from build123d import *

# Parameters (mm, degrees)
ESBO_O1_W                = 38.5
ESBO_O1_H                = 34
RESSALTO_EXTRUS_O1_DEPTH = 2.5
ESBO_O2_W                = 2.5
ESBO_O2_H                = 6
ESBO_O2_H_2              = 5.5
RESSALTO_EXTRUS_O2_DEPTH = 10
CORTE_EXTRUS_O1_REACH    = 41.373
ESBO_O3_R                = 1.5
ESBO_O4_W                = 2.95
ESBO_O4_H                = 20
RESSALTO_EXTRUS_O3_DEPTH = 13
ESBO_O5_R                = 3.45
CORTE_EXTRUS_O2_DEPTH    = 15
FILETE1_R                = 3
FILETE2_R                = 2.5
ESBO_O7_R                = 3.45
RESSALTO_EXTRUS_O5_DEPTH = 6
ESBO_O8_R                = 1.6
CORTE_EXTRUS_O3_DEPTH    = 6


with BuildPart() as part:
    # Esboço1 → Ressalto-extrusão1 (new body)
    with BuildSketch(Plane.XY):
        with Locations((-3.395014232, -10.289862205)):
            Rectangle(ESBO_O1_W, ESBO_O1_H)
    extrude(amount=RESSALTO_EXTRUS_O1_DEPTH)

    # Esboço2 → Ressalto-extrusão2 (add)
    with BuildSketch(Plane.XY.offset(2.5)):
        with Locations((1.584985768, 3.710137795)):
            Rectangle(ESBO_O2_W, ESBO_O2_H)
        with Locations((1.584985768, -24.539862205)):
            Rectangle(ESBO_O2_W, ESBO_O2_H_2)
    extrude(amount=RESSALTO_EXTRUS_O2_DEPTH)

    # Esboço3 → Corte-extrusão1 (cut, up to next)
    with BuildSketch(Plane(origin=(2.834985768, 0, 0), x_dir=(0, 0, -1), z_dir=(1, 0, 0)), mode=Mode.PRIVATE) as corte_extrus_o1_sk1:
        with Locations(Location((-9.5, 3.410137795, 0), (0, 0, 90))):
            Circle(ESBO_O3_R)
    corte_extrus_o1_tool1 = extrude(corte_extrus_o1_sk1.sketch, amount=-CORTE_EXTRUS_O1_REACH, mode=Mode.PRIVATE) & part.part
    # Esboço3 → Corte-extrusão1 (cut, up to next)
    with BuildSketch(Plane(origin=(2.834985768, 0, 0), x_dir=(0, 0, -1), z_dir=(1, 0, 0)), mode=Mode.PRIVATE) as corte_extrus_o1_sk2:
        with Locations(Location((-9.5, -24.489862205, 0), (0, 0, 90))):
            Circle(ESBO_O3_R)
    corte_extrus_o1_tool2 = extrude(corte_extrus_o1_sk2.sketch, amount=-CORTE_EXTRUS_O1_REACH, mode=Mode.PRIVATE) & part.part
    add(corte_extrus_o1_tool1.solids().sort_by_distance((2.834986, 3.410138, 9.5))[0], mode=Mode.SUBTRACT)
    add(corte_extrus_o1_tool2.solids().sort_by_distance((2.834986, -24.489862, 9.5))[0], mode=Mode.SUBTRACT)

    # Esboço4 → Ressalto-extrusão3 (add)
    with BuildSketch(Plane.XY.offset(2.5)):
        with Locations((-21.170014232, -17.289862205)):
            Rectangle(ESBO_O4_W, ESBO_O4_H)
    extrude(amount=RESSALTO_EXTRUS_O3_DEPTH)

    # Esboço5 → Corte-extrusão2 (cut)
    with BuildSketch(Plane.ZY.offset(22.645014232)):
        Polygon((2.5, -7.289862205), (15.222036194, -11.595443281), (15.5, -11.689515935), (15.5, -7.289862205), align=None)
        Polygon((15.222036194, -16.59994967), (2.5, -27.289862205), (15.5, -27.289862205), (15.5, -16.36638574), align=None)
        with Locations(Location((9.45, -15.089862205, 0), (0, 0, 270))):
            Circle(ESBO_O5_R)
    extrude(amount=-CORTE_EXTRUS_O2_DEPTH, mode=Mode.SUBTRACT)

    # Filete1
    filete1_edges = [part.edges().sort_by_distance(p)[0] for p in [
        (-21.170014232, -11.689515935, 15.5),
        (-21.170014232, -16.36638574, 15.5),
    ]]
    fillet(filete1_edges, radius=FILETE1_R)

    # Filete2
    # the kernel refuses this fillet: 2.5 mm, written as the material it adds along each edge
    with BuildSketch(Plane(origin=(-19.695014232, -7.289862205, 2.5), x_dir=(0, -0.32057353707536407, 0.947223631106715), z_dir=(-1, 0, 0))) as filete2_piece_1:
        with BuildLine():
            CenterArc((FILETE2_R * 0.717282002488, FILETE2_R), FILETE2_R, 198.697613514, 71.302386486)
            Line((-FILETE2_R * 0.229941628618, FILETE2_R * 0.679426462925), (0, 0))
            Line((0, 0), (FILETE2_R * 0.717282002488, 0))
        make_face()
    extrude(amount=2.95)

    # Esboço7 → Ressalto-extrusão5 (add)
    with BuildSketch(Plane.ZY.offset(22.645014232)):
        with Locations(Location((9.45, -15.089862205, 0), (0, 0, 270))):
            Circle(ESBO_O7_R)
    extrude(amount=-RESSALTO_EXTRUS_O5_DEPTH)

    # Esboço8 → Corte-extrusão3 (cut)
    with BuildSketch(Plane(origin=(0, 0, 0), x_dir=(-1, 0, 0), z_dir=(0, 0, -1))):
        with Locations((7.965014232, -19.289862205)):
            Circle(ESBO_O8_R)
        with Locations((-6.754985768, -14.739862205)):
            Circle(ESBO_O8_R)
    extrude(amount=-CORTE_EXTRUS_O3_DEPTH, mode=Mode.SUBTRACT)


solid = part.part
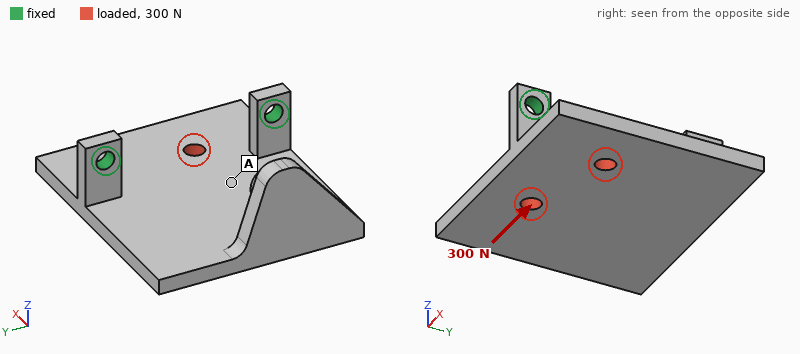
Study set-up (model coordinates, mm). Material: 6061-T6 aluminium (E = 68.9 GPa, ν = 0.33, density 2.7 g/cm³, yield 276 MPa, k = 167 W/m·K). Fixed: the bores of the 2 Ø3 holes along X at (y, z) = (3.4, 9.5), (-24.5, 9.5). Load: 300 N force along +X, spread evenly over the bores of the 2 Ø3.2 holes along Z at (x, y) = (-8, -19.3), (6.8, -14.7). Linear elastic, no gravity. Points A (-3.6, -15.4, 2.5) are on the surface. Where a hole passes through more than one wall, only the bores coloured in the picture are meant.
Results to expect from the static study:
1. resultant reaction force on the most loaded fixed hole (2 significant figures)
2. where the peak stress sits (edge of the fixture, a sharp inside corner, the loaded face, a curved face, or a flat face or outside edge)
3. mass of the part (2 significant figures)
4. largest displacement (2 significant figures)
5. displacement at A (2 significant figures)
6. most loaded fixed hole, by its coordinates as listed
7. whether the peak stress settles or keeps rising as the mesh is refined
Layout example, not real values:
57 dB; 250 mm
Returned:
220 N; edge of the fixture; 11 g; 0.20 mm; 0.053 mm; (-24.5, 9.5); keeps rising
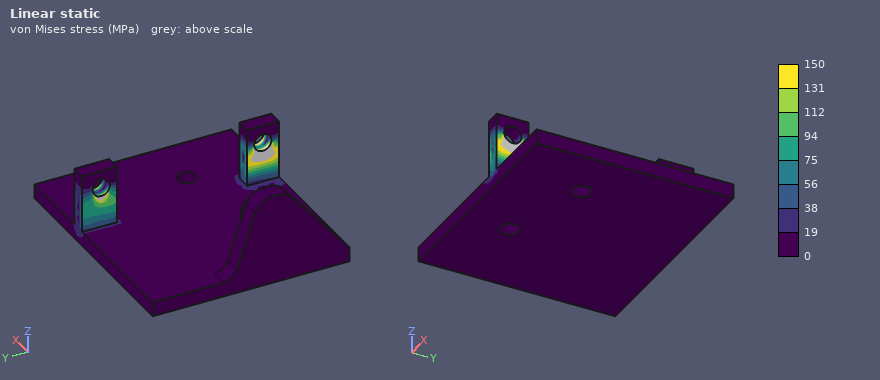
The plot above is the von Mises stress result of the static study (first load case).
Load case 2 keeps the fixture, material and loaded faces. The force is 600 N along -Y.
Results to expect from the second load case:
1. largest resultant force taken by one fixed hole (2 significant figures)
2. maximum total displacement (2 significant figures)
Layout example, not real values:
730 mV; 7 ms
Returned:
320 N; 37 µm
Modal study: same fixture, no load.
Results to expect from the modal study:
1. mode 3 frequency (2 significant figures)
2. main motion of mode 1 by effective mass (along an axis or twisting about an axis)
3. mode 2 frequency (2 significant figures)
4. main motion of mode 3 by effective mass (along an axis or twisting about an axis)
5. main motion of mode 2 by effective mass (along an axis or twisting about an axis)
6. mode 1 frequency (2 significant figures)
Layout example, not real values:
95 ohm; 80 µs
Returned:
4600 Hz; along Z; 3700 Hz; along X; along Y; 1200 Hz
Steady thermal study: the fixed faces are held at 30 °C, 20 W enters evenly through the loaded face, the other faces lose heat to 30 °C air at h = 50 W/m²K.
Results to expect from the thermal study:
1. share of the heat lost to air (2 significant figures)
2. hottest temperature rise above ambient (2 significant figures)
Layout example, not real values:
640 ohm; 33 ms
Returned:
24 %; 37 K
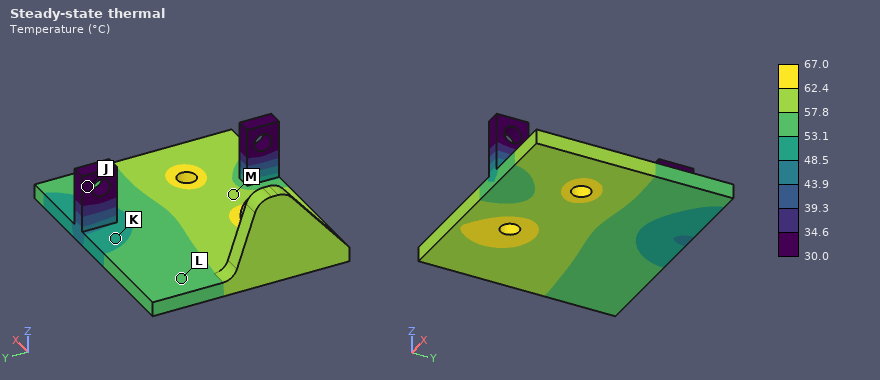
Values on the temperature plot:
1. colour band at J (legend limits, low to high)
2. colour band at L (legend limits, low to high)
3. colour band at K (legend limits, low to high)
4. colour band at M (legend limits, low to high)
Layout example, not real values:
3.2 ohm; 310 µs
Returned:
30.0 to 34.6 °C; 53.1 to 57.8 °C; 48.5 to 53.1 °C; 57.8 to 62.4 °C
